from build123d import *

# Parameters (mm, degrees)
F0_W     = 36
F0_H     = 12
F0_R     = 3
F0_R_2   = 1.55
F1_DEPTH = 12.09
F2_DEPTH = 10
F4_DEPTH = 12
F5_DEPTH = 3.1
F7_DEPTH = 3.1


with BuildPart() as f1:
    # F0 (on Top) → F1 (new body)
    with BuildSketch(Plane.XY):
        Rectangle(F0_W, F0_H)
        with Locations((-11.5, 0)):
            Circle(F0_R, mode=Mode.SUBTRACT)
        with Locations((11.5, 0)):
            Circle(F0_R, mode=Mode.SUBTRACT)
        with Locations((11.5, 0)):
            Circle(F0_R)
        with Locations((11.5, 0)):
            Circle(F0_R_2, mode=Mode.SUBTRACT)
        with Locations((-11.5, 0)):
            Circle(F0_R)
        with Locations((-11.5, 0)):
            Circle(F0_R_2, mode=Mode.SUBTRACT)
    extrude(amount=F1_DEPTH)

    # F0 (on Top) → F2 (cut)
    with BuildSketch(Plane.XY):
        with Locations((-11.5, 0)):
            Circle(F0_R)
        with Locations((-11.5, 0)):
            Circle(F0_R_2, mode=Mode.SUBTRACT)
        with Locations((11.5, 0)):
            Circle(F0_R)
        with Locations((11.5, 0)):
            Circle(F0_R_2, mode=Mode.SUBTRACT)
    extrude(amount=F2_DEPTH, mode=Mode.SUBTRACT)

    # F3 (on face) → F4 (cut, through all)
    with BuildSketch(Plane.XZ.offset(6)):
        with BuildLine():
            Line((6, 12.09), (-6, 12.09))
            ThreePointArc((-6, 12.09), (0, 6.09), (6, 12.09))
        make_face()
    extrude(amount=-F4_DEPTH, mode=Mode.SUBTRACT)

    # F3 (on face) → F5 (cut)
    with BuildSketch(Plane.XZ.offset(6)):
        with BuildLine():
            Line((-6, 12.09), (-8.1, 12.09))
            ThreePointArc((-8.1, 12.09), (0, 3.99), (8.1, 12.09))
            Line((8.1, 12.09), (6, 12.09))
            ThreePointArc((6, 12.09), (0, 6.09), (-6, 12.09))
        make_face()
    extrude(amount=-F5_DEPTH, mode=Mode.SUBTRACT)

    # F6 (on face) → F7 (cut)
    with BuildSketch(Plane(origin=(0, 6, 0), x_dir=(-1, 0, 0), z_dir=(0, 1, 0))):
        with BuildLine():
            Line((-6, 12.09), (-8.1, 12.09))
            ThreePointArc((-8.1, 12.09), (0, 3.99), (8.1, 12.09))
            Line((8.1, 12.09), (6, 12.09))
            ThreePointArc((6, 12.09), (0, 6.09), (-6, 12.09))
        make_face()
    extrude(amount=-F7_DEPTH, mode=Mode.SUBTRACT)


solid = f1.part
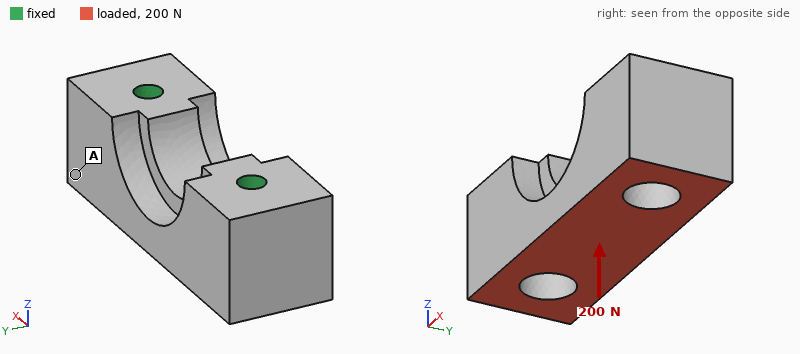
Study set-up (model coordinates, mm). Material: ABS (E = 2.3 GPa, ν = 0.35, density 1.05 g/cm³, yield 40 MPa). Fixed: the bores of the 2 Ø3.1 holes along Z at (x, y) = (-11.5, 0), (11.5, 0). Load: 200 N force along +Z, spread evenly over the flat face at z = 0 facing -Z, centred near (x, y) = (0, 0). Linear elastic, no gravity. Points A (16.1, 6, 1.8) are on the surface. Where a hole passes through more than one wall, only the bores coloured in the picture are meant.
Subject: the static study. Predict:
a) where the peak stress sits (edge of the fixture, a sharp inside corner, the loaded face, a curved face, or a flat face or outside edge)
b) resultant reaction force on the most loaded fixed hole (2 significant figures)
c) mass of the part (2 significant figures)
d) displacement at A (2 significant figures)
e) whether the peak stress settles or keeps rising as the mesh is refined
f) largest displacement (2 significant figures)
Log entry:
edge of the fixture
100 N
3.8 g
14 µm
keeps rising
23 µm
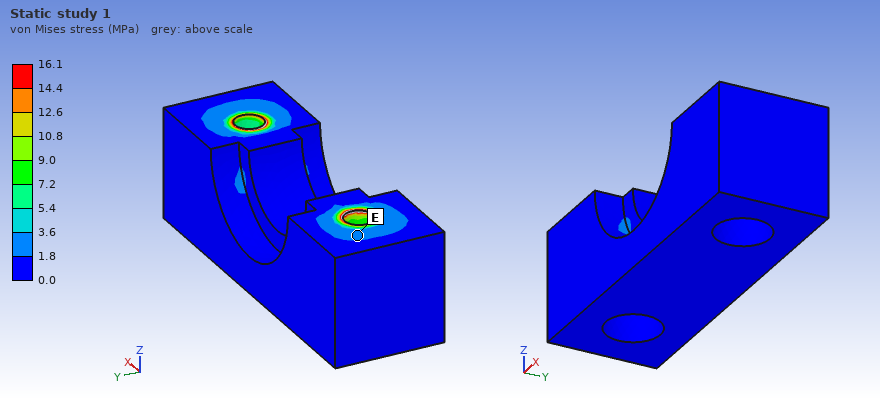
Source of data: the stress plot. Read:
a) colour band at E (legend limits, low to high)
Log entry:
1.8 to 3.6 MPa
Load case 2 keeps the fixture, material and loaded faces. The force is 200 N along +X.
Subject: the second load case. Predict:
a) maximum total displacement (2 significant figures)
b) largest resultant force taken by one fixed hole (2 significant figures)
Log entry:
68 µm
130 N
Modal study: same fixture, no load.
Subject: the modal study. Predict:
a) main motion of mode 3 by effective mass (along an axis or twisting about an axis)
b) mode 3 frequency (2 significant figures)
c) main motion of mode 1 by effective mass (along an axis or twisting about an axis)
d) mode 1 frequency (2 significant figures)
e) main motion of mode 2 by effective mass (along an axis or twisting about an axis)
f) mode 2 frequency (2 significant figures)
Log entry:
along X
6700 Hz
along Y
2700 Hz
twisting about Z
5000 Hz
